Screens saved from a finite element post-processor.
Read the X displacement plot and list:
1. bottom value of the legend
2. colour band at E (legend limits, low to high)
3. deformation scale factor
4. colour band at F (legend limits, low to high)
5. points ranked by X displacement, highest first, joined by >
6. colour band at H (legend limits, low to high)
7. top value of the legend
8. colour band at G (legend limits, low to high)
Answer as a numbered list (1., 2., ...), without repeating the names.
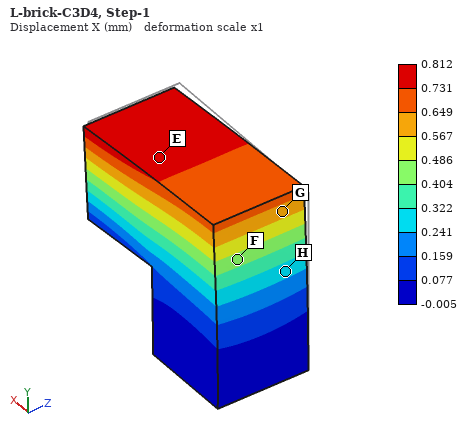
1. -0.005 mm
2. 0.731 to 0.812 mm
3. 1
4. 0.404 to 0.486 mm
5. E > G > F > H
6. 0.241 to 0.322 mm
7. 0.812 mm
8. 0.567 to 0.649 mm
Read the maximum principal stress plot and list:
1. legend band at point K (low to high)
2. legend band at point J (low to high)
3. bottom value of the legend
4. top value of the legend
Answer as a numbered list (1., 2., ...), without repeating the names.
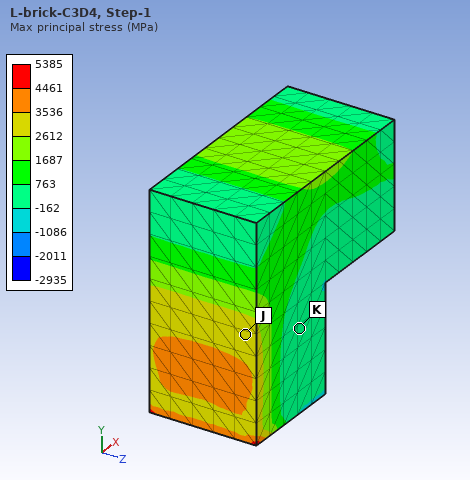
1. -162 to 763 MPa
2. 2612 to 3536 MPa
3. -2935 MPa
4. 5385 MPa
